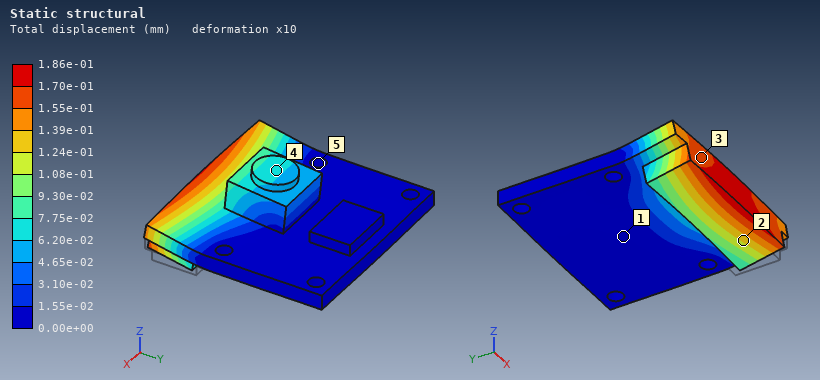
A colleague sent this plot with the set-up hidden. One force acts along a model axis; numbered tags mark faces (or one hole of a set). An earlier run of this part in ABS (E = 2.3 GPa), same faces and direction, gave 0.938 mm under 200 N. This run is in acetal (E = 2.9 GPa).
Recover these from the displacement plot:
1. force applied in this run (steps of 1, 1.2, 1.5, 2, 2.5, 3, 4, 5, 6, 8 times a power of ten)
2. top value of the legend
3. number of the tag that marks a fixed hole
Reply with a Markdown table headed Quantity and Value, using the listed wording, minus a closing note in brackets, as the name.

| Quantity | Value |
|---|---|
| force applied in this run | 50 N |
| top value of the legend | 1.86e-01 mm |
| number of the tag that marks a fixed hole | 5 |
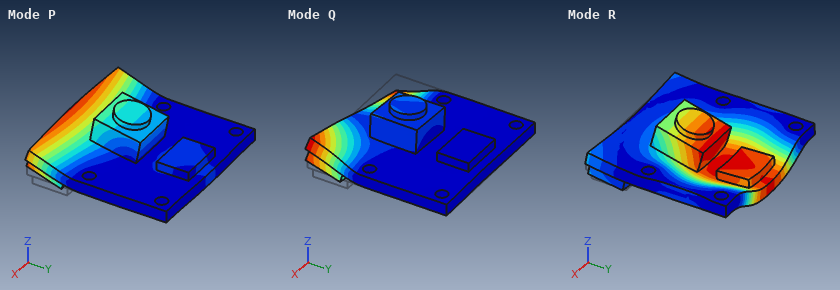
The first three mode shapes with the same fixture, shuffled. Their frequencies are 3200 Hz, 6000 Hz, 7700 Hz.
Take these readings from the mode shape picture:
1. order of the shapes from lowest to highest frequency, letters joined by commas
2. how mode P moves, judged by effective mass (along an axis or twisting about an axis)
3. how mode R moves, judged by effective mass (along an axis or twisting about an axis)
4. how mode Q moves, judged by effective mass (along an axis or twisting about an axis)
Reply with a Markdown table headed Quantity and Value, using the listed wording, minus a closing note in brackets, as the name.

| Quantity | Value |
|---|---|
| order of the shapes from lowest to highest frequency, letters joined by commas | P, R, Q |
| how mode P moves, judged by effective mass | along Z |
| how mode R moves, judged by effective mass | along Z |
| how mode Q moves, judged by effective mass | twisting about Y |
